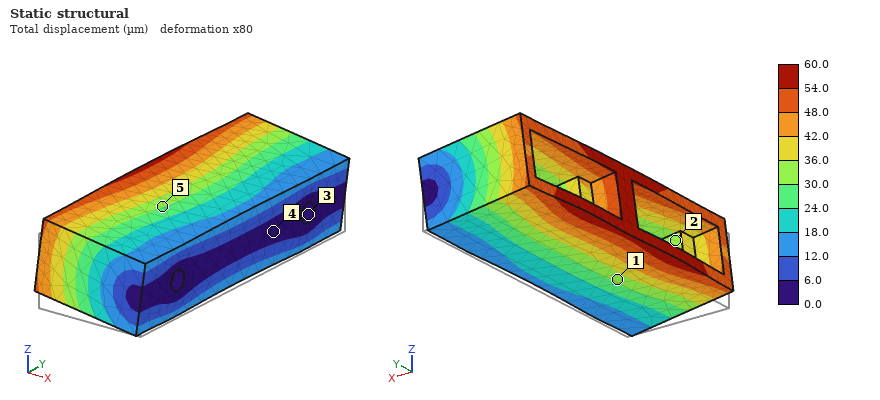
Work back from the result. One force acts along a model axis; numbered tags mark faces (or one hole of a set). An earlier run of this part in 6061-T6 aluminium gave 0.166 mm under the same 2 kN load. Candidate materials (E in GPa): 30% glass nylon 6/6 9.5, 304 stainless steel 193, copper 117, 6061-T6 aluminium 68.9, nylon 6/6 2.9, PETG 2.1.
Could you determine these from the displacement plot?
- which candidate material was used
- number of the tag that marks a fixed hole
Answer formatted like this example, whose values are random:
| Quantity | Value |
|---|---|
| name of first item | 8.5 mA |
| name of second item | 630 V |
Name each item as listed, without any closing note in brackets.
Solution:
| Quantity | Value |
|---|---|
| which candidate material was used | 304 stainless steel |
| number of the tag that marks a fixed hole | 3 |
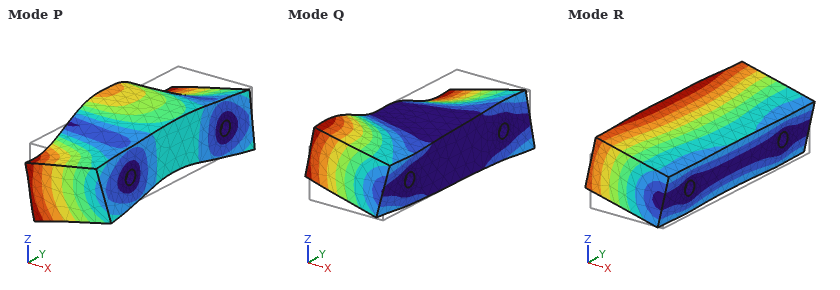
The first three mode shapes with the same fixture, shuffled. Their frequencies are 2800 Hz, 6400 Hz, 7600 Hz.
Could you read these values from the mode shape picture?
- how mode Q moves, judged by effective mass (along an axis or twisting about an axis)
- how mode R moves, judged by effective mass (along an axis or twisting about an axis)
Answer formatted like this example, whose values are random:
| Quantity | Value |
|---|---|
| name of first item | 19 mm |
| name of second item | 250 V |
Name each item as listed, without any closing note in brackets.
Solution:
| Quantity | Value |
|---|---|
| how mode Q moves, judged by effective mass | twisting about X |
| how mode R moves, judged by effective mass | along Z |
